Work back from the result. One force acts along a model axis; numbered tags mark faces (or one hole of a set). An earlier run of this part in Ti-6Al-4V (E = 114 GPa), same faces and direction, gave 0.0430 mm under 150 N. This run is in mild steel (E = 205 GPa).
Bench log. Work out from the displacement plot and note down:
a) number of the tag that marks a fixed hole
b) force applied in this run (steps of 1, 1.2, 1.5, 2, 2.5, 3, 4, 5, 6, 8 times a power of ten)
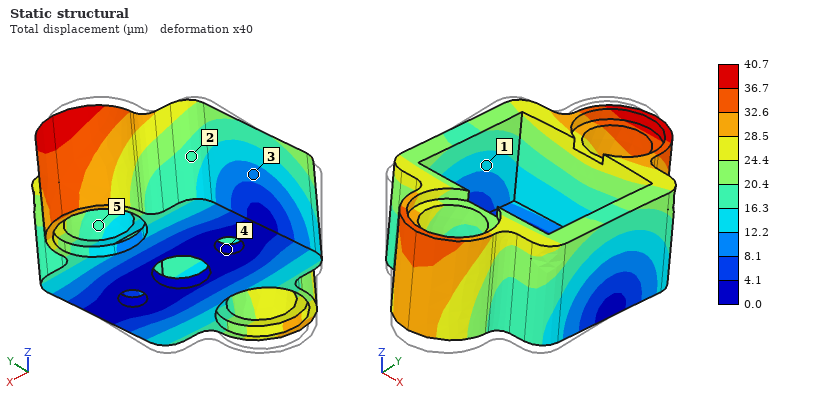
4
250 N
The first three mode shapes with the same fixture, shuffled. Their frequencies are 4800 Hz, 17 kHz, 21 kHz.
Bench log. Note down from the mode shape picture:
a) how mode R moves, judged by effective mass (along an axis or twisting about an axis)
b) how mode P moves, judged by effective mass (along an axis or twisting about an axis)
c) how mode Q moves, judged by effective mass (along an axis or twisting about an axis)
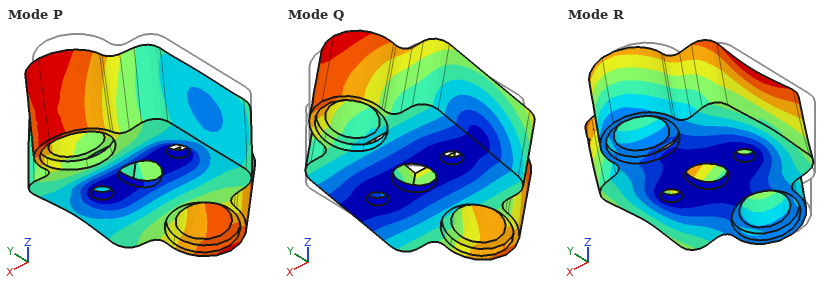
along X
along Z
along Y
